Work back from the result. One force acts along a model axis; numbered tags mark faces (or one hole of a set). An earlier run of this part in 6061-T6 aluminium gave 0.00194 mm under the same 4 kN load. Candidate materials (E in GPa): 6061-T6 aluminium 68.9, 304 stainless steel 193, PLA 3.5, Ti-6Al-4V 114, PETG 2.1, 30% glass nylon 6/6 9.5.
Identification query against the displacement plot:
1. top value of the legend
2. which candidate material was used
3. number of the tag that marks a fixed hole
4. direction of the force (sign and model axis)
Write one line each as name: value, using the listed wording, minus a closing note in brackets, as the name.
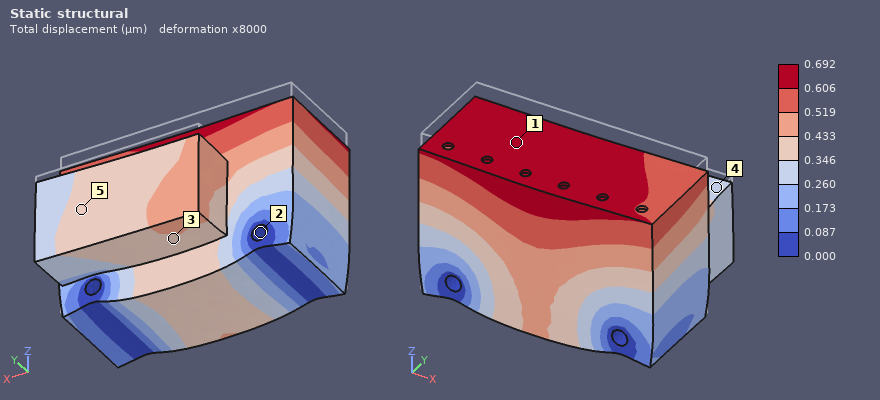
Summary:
top value of the legend: 0.692 µm
which candidate material was used: 304 stainless steel
number of the tag that marks a fixed hole: 2
direction of the force: -Z
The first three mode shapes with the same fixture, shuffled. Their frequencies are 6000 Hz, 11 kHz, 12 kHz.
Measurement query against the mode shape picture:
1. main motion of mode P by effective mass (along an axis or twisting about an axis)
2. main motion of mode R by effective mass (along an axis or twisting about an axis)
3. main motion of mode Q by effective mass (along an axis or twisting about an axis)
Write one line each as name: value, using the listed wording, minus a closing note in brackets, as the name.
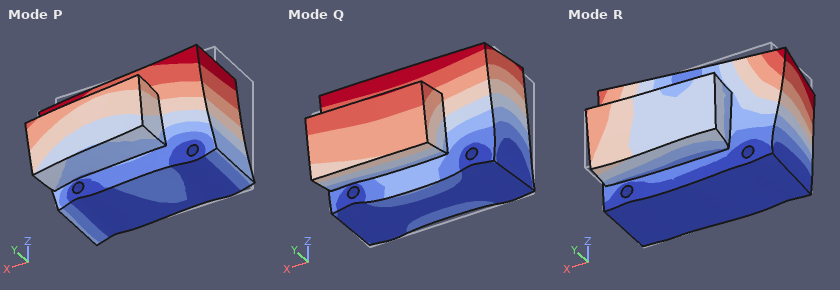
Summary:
main motion of mode P by effective mass: along X
main motion of mode R by effective mass: twisting about Z
main motion of mode Q by effective mass: along Y
